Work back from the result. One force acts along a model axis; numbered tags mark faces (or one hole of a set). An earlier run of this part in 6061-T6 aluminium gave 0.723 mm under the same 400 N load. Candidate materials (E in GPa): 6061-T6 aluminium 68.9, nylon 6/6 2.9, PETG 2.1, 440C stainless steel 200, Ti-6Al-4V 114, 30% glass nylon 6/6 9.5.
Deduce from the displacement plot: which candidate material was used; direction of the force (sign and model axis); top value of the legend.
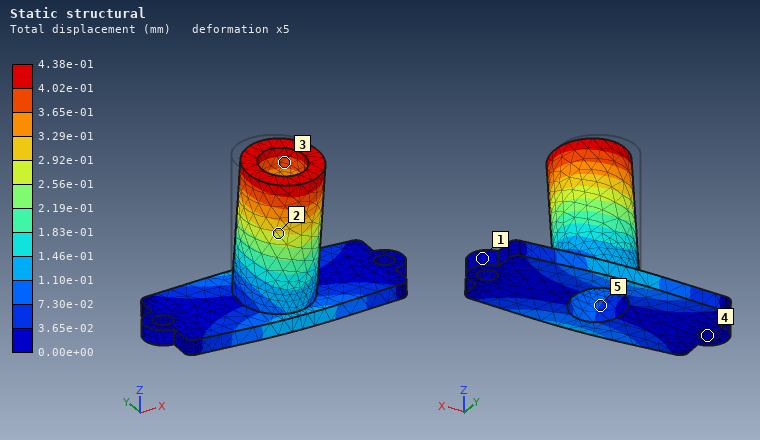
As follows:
Ti-6Al-4V
-Y
4.38e-01 mm
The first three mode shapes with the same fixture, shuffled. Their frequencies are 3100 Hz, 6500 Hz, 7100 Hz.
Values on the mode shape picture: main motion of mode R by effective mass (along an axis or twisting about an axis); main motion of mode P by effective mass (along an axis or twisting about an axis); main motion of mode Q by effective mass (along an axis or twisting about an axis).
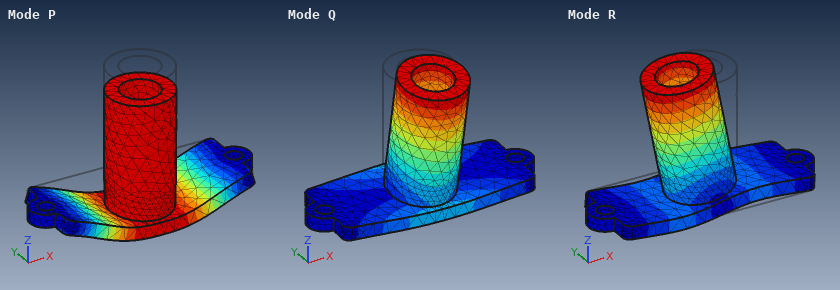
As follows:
along X
along Z
along Y
